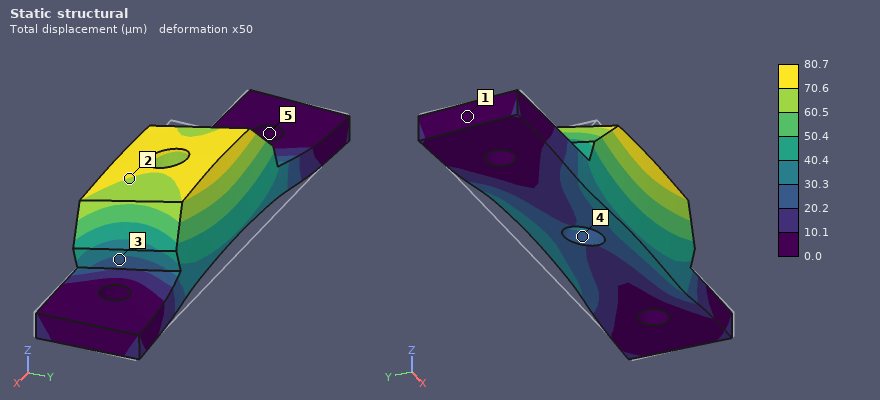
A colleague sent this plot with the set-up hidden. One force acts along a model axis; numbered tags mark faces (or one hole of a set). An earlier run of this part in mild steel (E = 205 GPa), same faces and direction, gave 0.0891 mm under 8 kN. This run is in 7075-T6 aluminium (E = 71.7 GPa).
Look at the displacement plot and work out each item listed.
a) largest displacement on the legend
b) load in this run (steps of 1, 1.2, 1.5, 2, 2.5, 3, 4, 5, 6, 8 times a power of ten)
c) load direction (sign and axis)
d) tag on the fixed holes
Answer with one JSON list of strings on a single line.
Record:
["80.7 µm", "2.5 kN", "-Y", "5"]
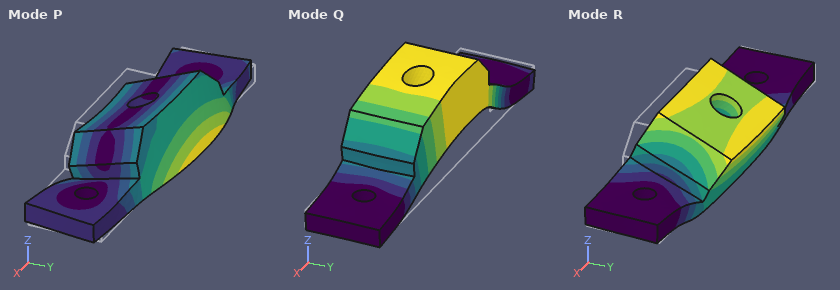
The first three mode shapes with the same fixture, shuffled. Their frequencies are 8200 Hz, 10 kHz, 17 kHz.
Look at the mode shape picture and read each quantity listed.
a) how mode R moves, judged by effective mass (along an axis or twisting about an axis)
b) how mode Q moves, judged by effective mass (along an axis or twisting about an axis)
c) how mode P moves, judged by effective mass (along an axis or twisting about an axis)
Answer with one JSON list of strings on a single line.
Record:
["along Y", "along Z", "along Y"]
